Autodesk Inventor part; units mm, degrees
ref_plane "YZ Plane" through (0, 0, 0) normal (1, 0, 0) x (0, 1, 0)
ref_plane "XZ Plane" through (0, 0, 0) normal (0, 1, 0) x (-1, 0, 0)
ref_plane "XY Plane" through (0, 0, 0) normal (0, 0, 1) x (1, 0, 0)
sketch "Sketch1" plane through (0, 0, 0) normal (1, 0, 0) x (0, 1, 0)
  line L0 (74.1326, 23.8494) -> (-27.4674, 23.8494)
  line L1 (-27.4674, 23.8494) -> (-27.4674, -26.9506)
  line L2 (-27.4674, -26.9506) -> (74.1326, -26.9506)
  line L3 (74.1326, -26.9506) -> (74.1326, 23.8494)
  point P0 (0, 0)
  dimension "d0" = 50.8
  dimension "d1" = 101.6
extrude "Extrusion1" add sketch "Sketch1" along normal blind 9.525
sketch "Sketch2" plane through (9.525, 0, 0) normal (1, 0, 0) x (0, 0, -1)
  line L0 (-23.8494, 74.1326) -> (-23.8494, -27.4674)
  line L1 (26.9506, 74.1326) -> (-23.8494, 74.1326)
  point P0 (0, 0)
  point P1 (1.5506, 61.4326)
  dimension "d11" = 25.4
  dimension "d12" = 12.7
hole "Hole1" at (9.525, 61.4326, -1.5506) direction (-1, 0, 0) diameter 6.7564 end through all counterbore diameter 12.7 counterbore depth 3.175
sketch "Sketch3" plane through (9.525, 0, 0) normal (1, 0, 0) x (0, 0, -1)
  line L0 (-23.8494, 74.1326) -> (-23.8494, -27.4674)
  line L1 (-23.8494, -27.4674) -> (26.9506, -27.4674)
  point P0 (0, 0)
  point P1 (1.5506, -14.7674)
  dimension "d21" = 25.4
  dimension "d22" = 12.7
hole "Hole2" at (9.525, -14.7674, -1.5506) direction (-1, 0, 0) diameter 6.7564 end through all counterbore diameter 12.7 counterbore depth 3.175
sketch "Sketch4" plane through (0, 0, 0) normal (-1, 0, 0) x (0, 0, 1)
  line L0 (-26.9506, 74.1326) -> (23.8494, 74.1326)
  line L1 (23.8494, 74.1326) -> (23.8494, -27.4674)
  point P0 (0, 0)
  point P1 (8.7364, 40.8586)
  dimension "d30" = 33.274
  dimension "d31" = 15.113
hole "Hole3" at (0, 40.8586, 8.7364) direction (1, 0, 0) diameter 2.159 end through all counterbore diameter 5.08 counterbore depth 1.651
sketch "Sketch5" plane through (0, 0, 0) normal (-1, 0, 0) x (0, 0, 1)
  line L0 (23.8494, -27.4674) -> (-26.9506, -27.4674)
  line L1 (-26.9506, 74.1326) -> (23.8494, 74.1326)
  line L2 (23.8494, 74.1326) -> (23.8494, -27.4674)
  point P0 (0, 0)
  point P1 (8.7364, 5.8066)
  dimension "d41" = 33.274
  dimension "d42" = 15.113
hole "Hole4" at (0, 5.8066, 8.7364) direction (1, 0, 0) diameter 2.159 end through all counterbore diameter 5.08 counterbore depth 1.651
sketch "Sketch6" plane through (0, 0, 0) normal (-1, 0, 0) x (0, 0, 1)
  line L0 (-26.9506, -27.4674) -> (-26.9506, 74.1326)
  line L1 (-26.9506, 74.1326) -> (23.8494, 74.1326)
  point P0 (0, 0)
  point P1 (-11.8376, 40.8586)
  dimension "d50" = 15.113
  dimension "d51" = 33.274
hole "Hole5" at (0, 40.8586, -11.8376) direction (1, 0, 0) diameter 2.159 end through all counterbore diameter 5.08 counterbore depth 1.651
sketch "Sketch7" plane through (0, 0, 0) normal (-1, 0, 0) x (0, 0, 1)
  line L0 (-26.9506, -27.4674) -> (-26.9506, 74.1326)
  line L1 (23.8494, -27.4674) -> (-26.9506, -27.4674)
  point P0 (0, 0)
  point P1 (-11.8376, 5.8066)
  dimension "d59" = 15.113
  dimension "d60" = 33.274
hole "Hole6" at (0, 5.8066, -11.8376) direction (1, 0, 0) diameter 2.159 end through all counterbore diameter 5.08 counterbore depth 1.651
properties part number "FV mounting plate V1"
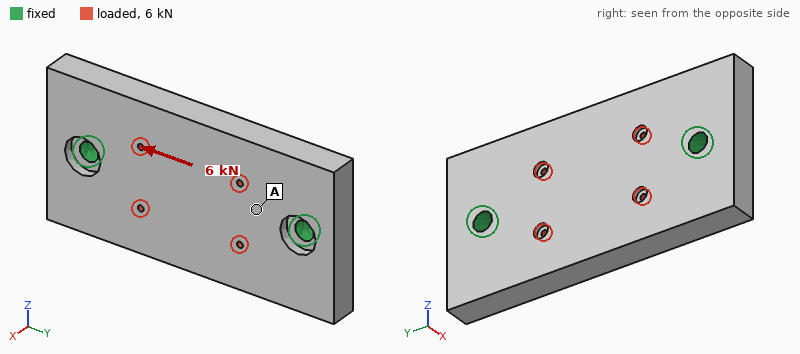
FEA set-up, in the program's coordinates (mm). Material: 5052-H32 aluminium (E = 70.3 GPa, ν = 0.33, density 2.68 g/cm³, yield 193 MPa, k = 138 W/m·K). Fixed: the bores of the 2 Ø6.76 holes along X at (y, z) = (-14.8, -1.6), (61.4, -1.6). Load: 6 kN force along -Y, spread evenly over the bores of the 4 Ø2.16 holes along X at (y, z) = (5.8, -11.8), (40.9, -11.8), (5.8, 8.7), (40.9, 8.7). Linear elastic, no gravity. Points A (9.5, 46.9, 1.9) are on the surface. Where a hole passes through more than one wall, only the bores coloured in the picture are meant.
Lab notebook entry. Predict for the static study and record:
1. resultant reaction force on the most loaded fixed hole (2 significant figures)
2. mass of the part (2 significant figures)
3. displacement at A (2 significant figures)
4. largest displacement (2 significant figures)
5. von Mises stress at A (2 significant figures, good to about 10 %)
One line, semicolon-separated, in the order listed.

3.0 kN; 130 g; 3.8 µm; 5.9 µm; 7.7 MPa
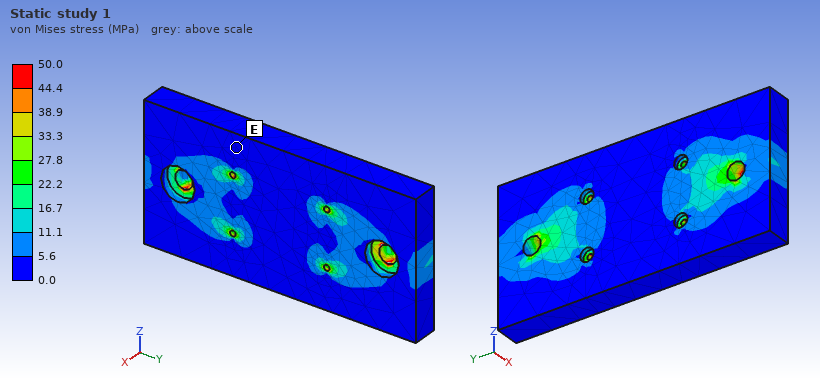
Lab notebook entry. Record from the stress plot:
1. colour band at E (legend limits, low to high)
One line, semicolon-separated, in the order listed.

0.0 to 5.6 MPa
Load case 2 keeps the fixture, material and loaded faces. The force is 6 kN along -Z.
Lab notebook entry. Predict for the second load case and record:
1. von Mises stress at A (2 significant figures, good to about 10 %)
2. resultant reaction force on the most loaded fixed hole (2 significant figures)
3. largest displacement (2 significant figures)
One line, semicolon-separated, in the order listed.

19 MPa; 3.0 kN; 22 µm
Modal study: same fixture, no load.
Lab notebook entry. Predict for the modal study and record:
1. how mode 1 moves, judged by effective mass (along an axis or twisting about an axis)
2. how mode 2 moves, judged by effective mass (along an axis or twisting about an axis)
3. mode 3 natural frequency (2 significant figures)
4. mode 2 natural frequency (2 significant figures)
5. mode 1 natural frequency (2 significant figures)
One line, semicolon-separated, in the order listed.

twisting about Y; along X; 8700 Hz; 5400 Hz; 4700 Hz
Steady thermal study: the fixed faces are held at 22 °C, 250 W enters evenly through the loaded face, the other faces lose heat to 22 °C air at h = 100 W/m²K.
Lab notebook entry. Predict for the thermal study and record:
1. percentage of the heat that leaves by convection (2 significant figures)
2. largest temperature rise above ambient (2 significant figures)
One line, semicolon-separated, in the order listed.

18 %; 65 K
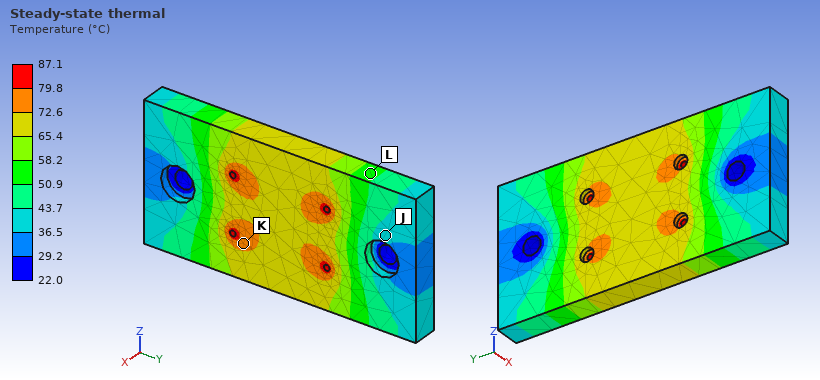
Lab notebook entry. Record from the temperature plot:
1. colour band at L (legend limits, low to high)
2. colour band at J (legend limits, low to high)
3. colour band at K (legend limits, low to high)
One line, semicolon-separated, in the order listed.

50.9 to 58.2 °C; 36.5 to 43.7 °C; 72.6 to 79.8 °C
